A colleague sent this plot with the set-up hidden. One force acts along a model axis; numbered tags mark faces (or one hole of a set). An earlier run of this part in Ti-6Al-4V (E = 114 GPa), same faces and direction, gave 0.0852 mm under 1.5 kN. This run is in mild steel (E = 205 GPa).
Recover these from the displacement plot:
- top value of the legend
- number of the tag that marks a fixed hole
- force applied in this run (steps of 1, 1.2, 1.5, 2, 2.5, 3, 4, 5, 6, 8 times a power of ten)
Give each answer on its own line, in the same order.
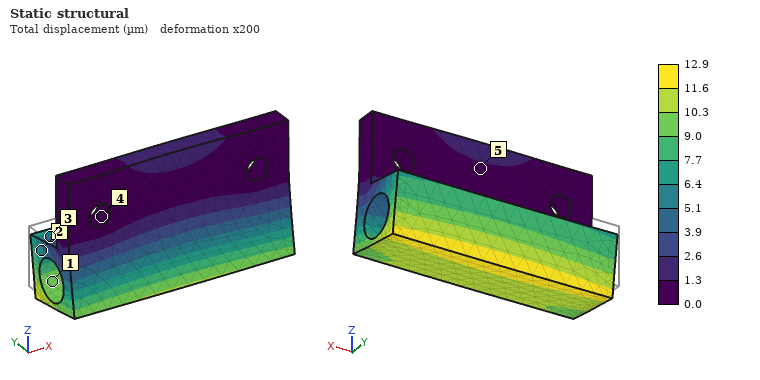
12.9 µm
4
400 N
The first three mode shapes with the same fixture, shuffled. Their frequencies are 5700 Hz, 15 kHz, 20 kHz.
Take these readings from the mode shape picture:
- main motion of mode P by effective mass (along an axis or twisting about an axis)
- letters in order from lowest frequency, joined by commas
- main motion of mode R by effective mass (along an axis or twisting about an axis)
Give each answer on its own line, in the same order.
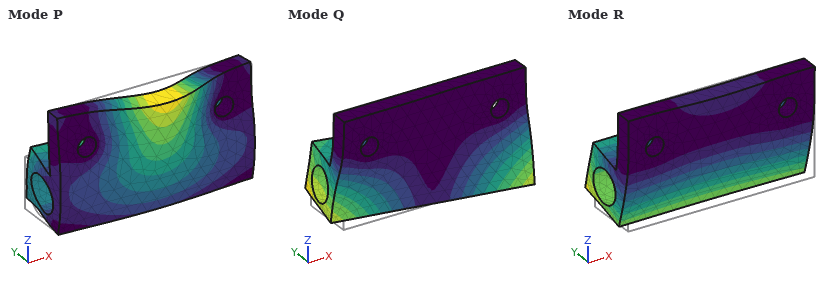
along Y
R, Q, P
along Y
